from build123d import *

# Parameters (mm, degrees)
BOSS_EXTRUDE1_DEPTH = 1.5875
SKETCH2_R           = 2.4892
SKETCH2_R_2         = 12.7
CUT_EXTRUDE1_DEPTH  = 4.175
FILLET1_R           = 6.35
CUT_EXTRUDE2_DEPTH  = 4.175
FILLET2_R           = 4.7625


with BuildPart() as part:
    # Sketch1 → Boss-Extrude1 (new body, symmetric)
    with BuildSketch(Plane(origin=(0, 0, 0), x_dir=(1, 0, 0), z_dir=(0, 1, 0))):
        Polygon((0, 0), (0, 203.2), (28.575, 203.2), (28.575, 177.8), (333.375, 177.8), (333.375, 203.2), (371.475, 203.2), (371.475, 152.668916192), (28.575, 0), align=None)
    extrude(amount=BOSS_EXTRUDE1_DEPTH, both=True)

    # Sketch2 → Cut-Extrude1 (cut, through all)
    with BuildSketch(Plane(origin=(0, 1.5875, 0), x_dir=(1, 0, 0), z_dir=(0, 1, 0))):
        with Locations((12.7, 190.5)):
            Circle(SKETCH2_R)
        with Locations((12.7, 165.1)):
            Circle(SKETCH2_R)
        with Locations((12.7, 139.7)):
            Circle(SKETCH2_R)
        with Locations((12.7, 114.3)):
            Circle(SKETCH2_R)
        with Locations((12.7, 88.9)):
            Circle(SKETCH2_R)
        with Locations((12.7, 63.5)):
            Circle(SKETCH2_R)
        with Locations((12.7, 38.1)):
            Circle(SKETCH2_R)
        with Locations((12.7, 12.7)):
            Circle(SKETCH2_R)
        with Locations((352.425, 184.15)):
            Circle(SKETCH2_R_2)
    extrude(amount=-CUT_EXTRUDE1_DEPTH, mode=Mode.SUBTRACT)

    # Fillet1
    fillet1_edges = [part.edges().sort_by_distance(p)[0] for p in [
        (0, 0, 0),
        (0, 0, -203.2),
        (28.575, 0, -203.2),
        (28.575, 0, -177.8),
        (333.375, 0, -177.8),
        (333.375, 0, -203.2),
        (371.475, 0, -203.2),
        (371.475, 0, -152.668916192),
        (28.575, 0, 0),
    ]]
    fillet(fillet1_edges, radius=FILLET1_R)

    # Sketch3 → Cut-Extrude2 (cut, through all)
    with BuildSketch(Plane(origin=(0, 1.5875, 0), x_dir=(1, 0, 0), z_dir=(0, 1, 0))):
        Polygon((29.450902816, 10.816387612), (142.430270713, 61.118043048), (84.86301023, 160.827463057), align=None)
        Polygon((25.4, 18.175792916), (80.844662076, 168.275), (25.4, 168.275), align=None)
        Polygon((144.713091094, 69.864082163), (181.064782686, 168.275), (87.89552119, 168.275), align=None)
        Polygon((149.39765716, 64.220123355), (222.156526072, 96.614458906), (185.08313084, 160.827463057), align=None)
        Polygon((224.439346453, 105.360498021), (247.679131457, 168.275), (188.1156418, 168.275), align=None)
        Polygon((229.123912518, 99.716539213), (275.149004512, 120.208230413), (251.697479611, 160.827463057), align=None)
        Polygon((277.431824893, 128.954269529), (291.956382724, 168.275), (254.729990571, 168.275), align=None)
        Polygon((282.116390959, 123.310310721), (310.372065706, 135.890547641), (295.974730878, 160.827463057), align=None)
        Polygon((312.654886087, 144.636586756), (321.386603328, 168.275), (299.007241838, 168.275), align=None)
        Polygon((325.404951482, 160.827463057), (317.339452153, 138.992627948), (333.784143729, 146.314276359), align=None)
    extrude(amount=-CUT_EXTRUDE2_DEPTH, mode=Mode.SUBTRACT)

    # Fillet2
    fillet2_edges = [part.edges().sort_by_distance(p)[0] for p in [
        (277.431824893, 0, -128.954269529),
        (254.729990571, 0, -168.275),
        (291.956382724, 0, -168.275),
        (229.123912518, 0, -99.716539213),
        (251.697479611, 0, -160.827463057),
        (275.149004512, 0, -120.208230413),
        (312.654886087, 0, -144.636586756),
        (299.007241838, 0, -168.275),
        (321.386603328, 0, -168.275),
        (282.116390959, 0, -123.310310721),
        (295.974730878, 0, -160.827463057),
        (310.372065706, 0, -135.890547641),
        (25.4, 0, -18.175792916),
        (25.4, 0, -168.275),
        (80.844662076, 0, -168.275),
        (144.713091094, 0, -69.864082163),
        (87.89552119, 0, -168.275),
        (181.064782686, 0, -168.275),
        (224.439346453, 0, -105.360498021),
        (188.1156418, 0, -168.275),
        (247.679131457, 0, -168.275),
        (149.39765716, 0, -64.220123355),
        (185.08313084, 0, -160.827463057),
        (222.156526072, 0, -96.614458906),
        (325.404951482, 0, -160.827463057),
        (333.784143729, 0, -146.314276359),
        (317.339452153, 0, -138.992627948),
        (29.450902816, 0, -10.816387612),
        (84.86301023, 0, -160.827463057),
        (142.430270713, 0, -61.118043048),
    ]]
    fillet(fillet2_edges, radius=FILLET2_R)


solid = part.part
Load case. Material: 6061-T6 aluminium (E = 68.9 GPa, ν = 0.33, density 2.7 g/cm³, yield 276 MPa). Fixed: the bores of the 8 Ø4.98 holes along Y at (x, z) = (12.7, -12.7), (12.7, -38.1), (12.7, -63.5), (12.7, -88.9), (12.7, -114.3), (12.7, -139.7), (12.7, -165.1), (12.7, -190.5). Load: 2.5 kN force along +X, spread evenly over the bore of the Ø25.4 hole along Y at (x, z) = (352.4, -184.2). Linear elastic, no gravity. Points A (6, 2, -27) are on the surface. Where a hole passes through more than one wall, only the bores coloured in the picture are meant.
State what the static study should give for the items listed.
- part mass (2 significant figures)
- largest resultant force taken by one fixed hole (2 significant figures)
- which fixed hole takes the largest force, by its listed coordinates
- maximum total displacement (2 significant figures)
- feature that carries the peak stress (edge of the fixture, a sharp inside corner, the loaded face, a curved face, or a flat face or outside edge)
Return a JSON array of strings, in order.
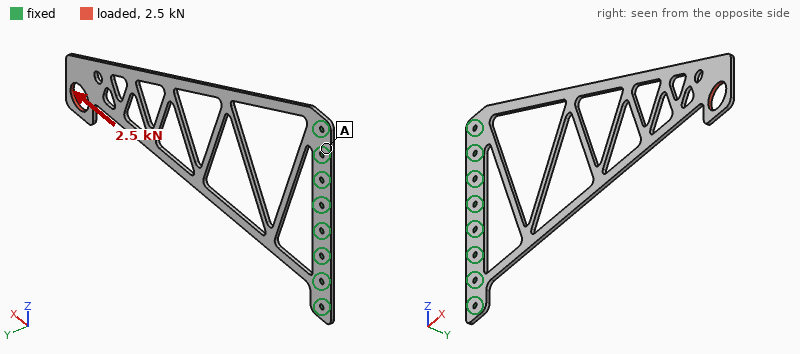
["150 g", "1.7 kN", "(12.7, -165.1)", "1.1 mm", "a curved face"]
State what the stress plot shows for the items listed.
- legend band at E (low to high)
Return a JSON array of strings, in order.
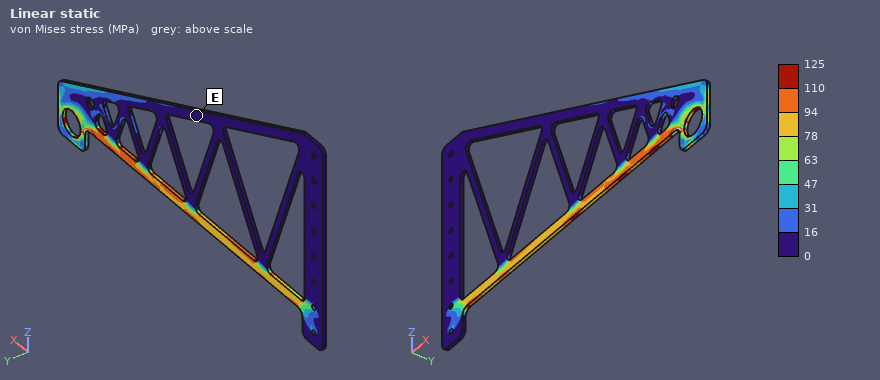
["0 to 16 MPa"]
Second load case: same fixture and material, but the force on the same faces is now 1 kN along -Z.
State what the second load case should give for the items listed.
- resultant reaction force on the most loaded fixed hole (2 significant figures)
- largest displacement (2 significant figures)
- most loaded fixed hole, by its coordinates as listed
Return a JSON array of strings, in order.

["2.7 kN", "1.2 mm", "(12.7, -12.7)"]
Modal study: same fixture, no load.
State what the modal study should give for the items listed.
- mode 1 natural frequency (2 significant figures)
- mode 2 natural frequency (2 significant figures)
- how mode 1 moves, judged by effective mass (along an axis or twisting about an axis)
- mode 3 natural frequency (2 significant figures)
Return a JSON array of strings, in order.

["16 Hz", "97 Hz", "along Y", "150 Hz"]
